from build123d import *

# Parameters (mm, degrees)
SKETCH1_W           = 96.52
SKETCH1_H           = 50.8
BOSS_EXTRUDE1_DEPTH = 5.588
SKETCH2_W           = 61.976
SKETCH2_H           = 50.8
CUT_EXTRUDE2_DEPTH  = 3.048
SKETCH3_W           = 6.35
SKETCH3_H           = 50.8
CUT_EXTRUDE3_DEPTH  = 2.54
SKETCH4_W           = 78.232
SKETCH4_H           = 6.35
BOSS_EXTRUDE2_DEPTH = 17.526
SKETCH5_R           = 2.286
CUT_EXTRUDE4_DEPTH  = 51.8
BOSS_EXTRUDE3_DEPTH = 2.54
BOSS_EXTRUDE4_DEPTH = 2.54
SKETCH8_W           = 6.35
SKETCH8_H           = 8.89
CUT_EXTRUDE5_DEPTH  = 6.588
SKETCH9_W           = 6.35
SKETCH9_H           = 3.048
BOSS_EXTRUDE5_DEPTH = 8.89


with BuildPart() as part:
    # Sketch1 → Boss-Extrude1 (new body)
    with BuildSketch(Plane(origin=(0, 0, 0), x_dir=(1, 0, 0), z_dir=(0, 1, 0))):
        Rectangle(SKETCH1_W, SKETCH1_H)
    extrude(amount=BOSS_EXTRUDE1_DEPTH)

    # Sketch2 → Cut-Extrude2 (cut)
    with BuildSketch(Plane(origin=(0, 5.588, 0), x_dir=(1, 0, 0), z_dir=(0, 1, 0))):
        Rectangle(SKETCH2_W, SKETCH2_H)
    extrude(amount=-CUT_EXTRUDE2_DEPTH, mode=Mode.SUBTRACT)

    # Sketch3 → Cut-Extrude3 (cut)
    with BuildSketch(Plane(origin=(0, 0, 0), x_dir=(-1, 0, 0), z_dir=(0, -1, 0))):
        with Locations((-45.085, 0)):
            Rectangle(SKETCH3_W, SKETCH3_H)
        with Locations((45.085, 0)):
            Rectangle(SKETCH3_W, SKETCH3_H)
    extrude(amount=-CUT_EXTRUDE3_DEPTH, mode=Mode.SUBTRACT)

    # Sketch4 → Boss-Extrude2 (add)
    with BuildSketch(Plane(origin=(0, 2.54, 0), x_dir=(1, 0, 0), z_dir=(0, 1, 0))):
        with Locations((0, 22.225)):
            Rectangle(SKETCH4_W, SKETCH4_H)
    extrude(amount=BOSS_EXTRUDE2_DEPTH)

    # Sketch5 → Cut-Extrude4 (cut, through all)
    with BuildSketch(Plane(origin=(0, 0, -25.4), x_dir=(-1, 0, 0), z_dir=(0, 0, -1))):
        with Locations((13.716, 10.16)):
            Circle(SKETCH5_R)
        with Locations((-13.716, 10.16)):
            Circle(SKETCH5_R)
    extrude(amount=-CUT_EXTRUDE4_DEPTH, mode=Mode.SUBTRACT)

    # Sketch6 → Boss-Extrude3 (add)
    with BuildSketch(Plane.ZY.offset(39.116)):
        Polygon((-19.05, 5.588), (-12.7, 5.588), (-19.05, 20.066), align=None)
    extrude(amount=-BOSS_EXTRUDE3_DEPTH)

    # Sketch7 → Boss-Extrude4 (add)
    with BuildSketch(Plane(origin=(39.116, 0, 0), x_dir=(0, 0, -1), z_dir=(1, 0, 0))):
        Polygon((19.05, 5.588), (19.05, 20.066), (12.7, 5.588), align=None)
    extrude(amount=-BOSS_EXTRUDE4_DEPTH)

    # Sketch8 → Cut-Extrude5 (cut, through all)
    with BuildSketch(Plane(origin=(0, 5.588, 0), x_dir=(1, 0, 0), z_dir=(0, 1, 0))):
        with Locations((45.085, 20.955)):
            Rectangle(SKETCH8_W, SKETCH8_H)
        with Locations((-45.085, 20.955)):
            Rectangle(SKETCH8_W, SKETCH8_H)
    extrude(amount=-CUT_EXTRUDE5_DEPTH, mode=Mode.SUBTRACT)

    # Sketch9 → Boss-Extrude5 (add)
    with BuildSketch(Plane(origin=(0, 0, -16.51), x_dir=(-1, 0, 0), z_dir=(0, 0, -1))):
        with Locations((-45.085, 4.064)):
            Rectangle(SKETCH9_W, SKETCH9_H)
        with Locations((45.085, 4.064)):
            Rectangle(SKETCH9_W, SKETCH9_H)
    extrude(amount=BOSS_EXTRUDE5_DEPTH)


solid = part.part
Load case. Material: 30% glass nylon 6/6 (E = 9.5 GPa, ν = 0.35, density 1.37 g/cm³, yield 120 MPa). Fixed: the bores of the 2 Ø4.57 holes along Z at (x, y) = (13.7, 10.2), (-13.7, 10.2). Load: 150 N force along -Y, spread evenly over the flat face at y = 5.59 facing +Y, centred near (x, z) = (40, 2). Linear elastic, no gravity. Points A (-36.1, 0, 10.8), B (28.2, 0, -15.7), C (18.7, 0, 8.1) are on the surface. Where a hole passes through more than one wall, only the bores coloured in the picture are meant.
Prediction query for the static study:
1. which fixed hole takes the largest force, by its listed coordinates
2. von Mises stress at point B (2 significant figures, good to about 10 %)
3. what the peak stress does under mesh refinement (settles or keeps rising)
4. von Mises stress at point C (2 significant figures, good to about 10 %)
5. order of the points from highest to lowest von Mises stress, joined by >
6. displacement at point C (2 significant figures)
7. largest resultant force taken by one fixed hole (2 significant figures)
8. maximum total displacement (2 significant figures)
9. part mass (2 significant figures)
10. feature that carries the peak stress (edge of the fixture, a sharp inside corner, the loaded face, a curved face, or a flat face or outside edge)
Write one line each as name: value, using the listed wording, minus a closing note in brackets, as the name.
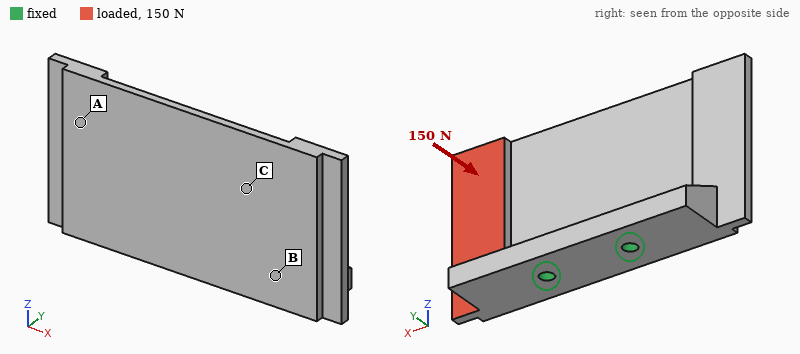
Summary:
which fixed hole takes the largest force, by its listed coordinates: (13.7, 10.2)
von Mises stress at point B: 13 MPa
what the peak stress does under mesh refinement: keeps rising
von Mises stress at point C: 6.7 MPa
order of the points from highest to lowest von Mises stress, joined by >: B > C > A
displacement at point C: 0.43 mm
largest resultant force taken by one fixed hole: 250 N
maximum total displacement: 1.2 mm
part mass: 34 g
feature that carries the peak stress: edge of the fixture
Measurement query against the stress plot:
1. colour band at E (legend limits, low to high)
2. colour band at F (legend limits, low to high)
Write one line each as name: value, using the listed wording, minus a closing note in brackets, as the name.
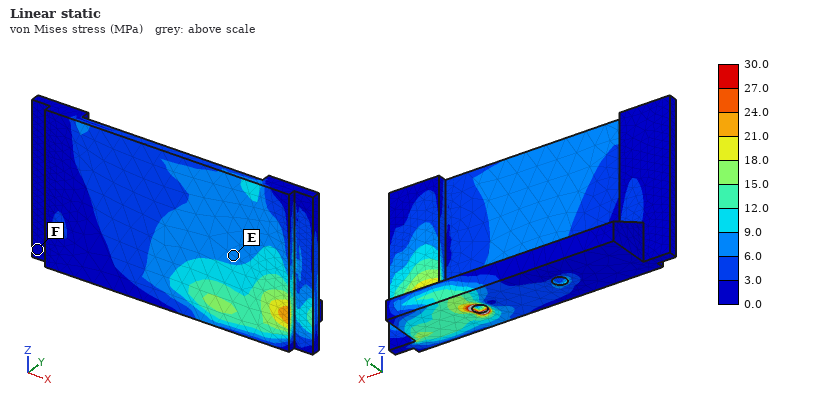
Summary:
colour band at E: 6.0 to 9.0 MPa
colour band at F: 0.0 to 3.0 MPa
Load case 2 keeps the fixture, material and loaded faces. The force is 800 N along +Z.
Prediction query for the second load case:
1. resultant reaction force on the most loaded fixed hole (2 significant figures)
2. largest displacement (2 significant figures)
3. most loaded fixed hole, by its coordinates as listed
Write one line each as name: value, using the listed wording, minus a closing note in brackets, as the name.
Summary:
resultant reaction force on the most loaded fixed hole: 1.3 kN
largest displacement: 0.70 mm
most loaded fixed hole, by its coordinates as listed: (13.7, 10.2)
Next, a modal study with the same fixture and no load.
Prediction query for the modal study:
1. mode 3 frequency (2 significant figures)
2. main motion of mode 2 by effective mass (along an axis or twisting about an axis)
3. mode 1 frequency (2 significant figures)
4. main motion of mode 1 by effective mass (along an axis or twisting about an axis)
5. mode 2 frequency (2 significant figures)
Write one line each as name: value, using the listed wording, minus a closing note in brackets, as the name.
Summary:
mode 3 frequency: 1700 Hz
main motion of mode 2 by effective mass: twisting about Z
mode 1 frequency: 720 Hz
main motion of mode 1 by effective mass: along Y
mode 2 frequency: 910 Hz
